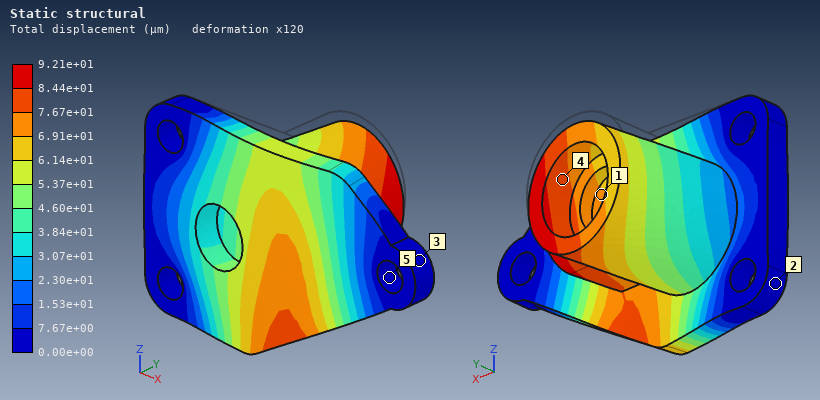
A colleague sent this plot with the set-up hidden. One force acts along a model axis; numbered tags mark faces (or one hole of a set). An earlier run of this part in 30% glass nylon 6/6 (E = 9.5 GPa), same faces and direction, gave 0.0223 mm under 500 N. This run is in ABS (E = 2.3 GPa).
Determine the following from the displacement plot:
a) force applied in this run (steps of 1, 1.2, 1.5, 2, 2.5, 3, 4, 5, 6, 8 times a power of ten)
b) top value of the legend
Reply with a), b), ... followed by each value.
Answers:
a) 500 N
b) 9.21e+01 µm
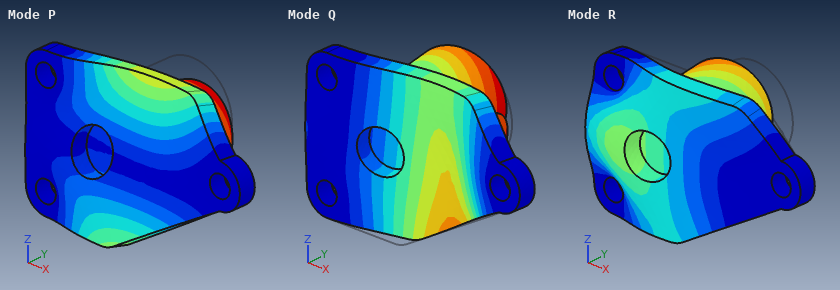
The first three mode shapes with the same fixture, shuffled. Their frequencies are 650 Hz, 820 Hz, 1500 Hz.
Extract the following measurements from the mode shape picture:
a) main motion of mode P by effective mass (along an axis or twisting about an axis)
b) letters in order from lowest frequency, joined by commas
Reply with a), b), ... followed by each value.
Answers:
a) along Z
b) Q, P, R
